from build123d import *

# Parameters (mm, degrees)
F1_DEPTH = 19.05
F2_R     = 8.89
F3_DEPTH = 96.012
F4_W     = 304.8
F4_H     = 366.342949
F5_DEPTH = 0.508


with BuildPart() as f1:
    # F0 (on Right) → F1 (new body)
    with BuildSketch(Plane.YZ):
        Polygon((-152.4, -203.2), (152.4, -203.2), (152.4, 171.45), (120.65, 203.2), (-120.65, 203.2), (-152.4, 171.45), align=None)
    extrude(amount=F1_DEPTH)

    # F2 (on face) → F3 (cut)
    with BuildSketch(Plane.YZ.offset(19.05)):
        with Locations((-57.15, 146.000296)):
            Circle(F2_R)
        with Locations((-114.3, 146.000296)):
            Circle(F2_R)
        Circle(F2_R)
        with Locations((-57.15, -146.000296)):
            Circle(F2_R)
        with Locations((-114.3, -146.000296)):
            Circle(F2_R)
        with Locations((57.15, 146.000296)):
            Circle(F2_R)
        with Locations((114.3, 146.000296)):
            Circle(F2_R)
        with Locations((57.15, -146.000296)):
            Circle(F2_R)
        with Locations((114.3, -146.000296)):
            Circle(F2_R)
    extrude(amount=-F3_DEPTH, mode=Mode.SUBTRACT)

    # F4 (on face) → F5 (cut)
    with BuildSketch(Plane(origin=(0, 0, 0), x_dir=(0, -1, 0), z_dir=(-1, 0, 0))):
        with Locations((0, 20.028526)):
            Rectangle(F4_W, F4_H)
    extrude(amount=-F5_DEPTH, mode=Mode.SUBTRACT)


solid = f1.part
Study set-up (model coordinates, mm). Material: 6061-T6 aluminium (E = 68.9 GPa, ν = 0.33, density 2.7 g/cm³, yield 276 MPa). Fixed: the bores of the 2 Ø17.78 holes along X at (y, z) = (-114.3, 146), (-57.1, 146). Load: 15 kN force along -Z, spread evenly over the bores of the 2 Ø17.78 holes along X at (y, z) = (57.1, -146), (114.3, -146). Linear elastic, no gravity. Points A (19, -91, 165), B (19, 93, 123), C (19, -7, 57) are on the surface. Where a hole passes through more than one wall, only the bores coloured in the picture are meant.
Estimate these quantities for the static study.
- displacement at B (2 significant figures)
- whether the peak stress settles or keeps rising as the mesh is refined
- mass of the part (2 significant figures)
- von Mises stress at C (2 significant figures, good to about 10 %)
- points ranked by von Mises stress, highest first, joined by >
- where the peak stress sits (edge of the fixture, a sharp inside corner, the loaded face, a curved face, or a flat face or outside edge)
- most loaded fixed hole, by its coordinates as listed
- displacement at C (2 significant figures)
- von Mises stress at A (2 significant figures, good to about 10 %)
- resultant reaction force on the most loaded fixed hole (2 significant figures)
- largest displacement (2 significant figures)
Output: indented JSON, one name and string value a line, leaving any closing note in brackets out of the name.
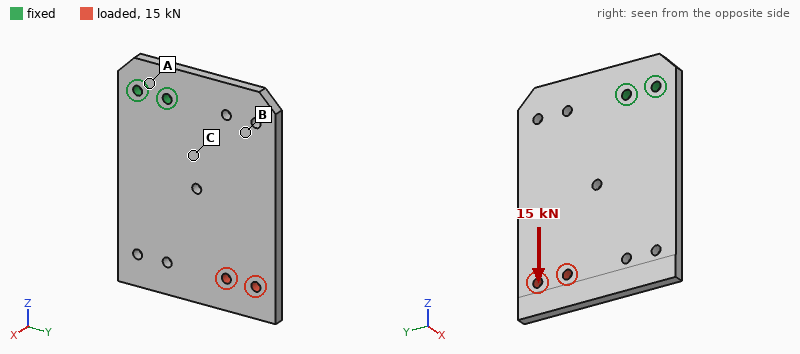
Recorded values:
{
  "displacement at B": "0.15 mm",
  "whether the peak stress settles or keeps rising as the mesh is refined": "keeps rising",
  "mass of the part": "6.1 kg",
  "von Mises stress at C": "9.1 MPa",
  "points ranked by von Mises stress, highest first, joined by >": "A > C > B",
  "where the peak stress sits": "edge of the fixture",
  "most loaded fixed hole, by its coordinates as listed": "(-57.1, 146)",
  "displacement at C": "0.094 mm",
  "von Mises stress at A": "19 MPa",
  "resultant reaction force on the most loaded fixed hole": "44 kN",
  "largest displacement": "0.37 mm"
}
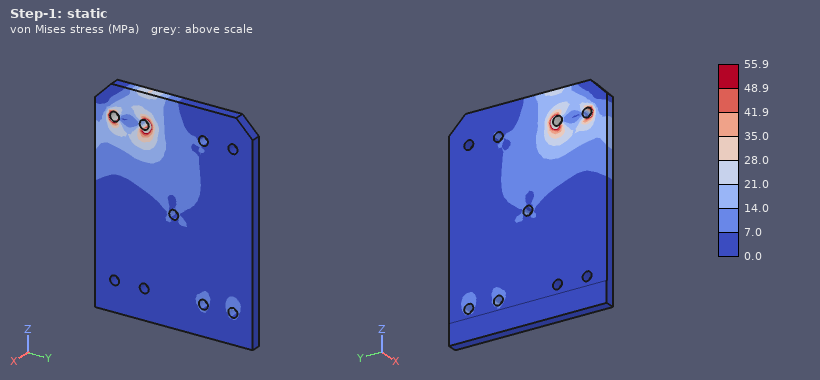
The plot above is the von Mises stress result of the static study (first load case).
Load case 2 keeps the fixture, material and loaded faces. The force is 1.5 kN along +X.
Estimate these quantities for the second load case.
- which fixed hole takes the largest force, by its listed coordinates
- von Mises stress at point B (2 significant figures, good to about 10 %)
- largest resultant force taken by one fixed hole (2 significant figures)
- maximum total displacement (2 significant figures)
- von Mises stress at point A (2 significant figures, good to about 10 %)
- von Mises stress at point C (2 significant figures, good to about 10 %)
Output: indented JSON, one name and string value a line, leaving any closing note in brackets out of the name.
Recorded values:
{
  "which fixed hole takes the largest force, by its listed coordinates": "(-57.1, 146)",
  "von Mises stress at point B": "14 MPa",
  "largest resultant force taken by one fixed hole": "3.3 kN",
  "maximum total displacement": "2.7 mm",
  "von Mises stress at point A": "7.6 MPa",
  "von Mises stress at point C": "18 MPa"
}
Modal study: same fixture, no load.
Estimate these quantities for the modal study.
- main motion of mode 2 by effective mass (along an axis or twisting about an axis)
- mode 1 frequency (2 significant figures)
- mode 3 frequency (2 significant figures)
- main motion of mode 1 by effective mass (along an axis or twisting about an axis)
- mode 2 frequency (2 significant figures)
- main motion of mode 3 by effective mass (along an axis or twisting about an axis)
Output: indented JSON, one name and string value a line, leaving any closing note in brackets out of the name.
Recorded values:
{
  "main motion of mode 2 by effective mass": "twisting about Z",
  "mode 1 frequency": "100 Hz",
  "mode 3 frequency": "480 Hz",
  "main motion of mode 1 by effective mass": "along X",
  "mode 2 frequency": "230 Hz",
  "main motion of mode 3 by effective mass": "along X"
}
